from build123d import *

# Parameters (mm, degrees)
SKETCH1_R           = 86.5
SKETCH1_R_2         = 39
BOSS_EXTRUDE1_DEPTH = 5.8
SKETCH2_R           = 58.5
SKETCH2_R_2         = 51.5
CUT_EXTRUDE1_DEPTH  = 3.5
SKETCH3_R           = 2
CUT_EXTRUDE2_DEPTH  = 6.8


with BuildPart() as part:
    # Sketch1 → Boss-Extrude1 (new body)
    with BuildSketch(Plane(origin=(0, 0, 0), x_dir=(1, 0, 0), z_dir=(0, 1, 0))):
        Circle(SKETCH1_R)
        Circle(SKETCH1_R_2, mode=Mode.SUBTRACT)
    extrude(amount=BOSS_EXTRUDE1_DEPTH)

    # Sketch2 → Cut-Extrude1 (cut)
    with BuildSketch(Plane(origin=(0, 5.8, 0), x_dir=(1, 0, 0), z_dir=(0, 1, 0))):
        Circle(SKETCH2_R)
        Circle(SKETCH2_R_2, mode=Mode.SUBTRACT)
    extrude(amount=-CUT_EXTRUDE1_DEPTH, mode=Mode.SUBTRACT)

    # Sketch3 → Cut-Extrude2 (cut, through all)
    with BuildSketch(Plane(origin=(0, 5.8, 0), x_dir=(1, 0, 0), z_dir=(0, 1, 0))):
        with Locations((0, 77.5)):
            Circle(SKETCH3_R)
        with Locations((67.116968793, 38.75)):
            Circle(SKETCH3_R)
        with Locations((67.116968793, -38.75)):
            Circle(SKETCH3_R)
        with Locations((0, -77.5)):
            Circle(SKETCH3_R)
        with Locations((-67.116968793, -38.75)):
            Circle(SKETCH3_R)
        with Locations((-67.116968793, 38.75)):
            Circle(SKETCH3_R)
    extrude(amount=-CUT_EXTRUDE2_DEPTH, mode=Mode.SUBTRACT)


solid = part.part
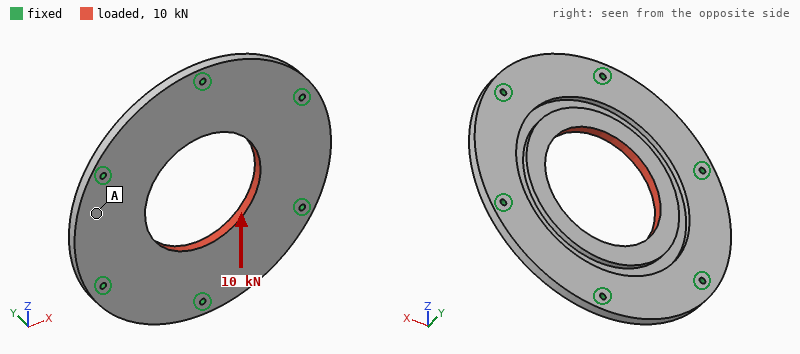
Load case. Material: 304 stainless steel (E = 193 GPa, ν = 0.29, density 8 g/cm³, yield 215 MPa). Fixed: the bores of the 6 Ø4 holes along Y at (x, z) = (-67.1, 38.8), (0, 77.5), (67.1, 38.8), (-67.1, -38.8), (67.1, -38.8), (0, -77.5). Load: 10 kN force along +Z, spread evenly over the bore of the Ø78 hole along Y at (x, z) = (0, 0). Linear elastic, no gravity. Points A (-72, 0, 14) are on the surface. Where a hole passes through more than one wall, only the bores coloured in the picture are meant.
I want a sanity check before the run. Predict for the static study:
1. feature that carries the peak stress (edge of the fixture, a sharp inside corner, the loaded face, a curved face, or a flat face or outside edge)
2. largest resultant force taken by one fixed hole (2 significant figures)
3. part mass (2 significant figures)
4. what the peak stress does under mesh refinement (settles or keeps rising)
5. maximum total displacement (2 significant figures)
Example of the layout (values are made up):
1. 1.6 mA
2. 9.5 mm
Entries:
1. edge of the fixture
2. 2.0 kN
3. 800 g
4. keeps rising
5. 7.8 µm
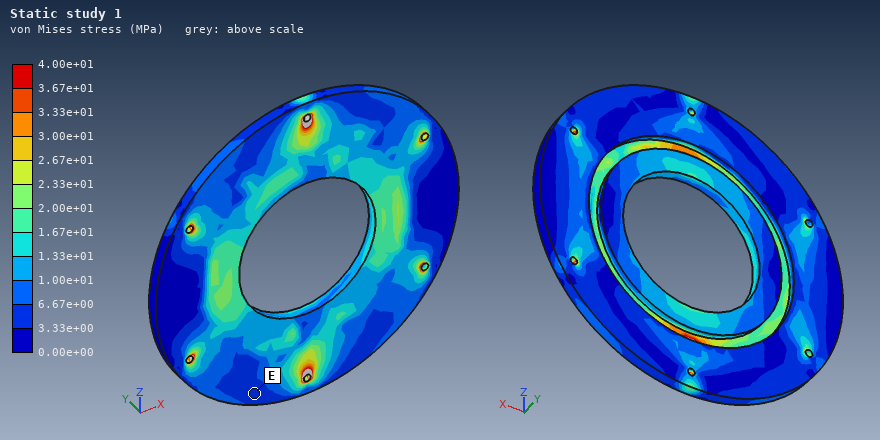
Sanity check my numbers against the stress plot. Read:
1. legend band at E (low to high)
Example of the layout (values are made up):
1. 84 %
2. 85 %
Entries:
1. 3.33e+00 to 6.67e+00 MPa
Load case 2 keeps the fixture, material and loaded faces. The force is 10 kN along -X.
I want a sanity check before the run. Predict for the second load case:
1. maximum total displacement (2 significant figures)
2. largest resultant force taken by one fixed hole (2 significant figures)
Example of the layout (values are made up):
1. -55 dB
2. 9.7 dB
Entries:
1. 7.9 µm
2. 1.9 kN
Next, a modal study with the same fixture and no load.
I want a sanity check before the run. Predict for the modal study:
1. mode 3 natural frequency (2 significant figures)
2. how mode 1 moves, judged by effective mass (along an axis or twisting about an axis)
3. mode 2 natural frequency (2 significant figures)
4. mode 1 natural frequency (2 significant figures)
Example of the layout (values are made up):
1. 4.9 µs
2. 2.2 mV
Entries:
1. 3400 Hz
2. along Y
3. 3400 Hz
4. 2600 Hz
